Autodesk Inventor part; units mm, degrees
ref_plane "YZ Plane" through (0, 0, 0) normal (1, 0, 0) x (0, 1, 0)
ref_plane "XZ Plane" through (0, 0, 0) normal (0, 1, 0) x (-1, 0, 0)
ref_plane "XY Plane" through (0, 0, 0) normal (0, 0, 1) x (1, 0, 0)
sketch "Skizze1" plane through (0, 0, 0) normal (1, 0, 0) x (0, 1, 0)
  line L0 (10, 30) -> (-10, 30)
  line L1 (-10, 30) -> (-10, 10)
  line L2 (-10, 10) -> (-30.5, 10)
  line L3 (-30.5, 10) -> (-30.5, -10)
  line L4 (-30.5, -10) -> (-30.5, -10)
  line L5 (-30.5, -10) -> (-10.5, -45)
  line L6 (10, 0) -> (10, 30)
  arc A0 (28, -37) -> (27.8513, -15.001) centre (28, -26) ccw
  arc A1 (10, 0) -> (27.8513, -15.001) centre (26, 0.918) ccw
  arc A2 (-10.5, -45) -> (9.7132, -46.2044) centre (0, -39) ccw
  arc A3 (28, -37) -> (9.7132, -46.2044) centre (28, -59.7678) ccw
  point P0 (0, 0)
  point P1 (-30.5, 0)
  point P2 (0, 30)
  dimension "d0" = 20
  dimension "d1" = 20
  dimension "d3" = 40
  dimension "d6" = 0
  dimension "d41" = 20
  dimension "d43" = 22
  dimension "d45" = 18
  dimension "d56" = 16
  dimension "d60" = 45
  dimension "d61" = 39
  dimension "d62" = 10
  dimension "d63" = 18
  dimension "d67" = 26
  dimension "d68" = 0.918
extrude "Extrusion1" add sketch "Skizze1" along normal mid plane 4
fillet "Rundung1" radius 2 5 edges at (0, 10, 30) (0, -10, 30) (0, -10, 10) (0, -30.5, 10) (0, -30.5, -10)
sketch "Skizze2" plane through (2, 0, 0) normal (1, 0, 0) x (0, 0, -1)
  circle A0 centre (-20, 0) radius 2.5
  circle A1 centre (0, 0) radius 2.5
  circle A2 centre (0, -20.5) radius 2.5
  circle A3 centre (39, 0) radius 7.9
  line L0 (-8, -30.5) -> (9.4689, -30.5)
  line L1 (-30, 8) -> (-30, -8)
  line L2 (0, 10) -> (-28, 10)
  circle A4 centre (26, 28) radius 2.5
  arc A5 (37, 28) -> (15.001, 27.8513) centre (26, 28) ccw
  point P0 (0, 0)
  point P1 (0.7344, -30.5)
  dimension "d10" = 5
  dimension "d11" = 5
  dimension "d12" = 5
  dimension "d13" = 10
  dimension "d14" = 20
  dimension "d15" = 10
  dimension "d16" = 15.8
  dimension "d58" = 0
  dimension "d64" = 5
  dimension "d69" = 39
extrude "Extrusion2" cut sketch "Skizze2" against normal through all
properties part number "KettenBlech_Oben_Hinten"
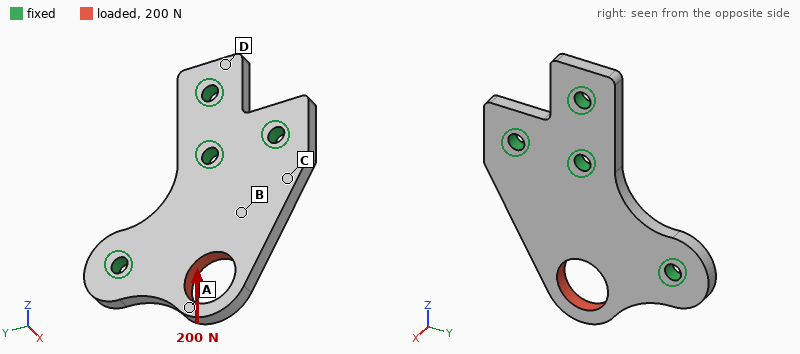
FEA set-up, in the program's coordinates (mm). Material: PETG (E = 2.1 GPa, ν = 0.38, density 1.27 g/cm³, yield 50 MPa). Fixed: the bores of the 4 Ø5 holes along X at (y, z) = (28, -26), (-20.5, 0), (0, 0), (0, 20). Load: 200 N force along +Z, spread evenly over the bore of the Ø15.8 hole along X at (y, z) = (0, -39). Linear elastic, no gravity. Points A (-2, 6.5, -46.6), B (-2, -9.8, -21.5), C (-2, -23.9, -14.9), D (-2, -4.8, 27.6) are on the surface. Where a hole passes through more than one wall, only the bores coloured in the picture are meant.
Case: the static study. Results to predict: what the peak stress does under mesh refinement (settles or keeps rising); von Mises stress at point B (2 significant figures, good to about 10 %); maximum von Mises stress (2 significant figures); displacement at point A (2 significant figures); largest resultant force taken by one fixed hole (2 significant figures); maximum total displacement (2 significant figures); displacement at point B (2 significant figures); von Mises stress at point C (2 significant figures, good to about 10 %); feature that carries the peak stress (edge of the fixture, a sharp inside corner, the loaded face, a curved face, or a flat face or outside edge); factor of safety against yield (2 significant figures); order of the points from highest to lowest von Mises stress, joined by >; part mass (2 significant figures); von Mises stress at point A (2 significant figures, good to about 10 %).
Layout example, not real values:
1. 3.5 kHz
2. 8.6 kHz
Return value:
1. settles
2. 1.3 MPa
3. 5.0 MPa
4. 43 µm
5. 79 N
6. 54 µm
7. 13 µm
8. 0.80 MPa
9. the loaded face
10. 10
11. A > B > C > D
12. 14 g
13. 2.3 MPa
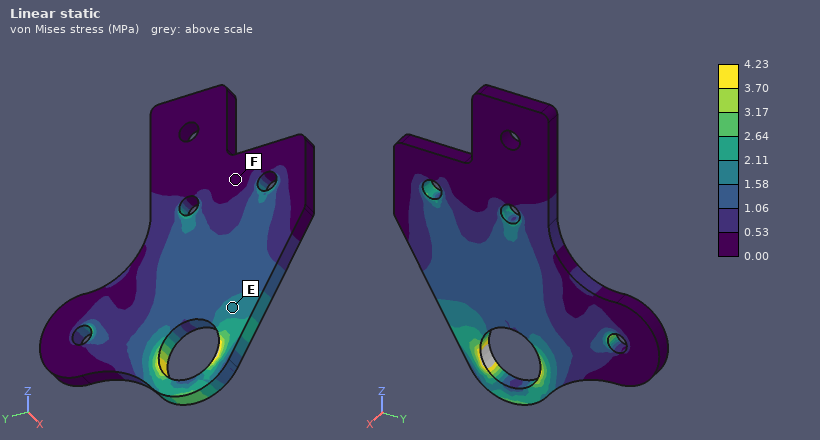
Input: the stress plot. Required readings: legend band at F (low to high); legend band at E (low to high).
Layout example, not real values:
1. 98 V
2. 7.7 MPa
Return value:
1. 0.00 to 0.53 MPa
2. 1.58 to 2.11 MPa
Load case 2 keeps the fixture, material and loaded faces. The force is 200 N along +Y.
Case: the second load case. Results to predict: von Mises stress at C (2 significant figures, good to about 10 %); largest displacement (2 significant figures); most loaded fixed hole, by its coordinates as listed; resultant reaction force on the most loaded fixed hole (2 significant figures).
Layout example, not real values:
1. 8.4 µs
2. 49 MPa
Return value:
1. 1.3 MPa
2. 0.11 mm
3. (28, -26)
4. 170 N
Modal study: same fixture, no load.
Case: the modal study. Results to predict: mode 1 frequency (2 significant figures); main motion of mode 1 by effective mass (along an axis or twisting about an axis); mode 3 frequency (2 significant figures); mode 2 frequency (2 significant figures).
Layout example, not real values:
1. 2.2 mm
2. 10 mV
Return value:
1. 850 Hz
2. along X
3. 2900 Hz
4. 2000 Hz
